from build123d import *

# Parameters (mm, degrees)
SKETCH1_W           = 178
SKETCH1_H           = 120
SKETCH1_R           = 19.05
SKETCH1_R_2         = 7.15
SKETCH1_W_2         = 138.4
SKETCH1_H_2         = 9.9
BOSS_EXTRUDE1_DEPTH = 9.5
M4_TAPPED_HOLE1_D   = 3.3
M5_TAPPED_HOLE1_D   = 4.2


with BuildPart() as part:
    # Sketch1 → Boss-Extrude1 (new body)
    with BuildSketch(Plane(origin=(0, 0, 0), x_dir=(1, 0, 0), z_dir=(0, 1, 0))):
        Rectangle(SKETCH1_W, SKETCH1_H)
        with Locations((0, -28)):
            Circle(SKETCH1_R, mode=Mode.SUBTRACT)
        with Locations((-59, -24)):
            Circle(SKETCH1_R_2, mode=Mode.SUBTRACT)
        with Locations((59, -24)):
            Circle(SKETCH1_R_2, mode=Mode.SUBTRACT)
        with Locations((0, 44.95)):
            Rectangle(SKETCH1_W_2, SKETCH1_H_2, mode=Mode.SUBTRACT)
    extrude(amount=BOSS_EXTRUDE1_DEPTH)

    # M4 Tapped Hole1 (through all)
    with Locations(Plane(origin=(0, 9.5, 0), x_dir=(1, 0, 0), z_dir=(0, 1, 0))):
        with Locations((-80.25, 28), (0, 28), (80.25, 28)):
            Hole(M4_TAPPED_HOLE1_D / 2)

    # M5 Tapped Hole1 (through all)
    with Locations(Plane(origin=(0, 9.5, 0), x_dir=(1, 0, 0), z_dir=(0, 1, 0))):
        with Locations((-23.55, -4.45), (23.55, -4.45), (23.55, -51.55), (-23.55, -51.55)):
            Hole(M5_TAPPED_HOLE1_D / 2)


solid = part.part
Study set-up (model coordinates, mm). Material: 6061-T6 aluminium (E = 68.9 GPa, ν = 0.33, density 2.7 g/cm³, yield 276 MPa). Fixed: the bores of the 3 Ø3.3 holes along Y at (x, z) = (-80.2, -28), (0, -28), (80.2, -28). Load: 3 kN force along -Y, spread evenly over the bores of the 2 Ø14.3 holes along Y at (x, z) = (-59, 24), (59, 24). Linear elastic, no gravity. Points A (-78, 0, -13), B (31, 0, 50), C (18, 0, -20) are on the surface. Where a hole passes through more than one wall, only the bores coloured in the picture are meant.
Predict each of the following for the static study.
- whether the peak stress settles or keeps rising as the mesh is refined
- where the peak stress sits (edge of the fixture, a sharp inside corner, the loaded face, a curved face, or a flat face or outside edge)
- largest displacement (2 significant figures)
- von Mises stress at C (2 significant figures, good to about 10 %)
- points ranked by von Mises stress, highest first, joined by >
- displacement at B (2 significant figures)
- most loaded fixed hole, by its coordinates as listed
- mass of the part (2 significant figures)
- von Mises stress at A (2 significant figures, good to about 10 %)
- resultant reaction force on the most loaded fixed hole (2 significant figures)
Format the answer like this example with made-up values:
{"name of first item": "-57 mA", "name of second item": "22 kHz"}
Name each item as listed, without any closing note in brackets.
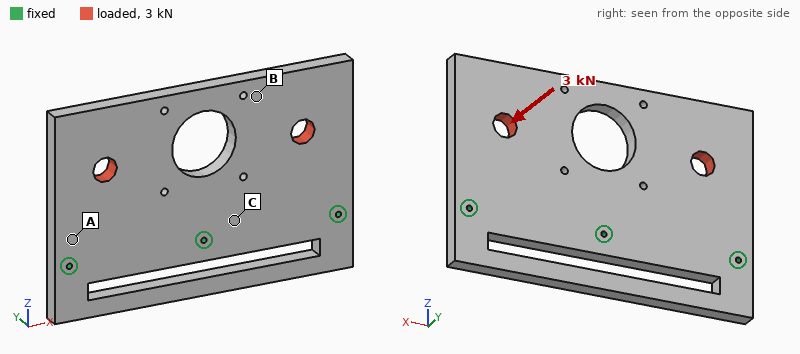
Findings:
{"whether the peak stress settles or keeps rising as the mesh is refined": "keeps rising", "where the peak stress sits": "edge of the fixture", "largest displacement": "0.65 mm", "von Mises stress at C": "34 MPa", "points ranked by von Mises stress, highest first, joined by >": "A > C > B", "displacement at B": "0.55 mm", "most loaded fixed hole, by its coordinates as listed": "(0, -28)", "mass of the part": "470 g", "von Mises stress at A": "60 MPa", "resultant reaction force on the most loaded fixed hole": "1.1 kN"}
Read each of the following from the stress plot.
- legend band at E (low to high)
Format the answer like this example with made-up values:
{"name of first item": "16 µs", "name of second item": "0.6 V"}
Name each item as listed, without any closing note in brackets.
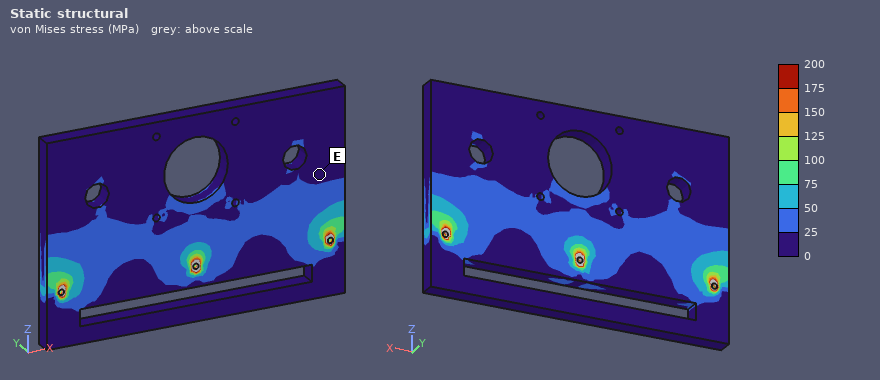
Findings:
{"legend band at E": "0 to 25 MPa"}
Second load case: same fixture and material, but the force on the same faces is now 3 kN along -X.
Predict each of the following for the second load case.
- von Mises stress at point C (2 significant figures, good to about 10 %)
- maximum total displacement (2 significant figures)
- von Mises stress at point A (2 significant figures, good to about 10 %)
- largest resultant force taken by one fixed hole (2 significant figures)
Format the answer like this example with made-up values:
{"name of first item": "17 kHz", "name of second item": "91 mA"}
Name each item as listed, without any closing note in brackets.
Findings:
{"von Mises stress at point C": "3.5 MPa", "maximum total displacement": "8.7 µm", "von Mises stress at point A": "4.4 MPa", "largest resultant force taken by one fixed hole": "1.4 kN"}
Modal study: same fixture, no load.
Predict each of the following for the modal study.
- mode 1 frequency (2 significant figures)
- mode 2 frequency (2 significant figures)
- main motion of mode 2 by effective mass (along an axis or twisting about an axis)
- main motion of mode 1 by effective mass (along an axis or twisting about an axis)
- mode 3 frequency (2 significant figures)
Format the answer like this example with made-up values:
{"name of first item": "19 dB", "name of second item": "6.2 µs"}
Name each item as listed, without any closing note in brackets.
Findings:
{"mode 1 frequency": "760 Hz", "mode 2 frequency": "1300 Hz", "main motion of mode 2 by effective mass": "twisting about Z", "main motion of mode 1 by effective mass": "along Y", "mode 3 frequency": "1600 Hz"}
